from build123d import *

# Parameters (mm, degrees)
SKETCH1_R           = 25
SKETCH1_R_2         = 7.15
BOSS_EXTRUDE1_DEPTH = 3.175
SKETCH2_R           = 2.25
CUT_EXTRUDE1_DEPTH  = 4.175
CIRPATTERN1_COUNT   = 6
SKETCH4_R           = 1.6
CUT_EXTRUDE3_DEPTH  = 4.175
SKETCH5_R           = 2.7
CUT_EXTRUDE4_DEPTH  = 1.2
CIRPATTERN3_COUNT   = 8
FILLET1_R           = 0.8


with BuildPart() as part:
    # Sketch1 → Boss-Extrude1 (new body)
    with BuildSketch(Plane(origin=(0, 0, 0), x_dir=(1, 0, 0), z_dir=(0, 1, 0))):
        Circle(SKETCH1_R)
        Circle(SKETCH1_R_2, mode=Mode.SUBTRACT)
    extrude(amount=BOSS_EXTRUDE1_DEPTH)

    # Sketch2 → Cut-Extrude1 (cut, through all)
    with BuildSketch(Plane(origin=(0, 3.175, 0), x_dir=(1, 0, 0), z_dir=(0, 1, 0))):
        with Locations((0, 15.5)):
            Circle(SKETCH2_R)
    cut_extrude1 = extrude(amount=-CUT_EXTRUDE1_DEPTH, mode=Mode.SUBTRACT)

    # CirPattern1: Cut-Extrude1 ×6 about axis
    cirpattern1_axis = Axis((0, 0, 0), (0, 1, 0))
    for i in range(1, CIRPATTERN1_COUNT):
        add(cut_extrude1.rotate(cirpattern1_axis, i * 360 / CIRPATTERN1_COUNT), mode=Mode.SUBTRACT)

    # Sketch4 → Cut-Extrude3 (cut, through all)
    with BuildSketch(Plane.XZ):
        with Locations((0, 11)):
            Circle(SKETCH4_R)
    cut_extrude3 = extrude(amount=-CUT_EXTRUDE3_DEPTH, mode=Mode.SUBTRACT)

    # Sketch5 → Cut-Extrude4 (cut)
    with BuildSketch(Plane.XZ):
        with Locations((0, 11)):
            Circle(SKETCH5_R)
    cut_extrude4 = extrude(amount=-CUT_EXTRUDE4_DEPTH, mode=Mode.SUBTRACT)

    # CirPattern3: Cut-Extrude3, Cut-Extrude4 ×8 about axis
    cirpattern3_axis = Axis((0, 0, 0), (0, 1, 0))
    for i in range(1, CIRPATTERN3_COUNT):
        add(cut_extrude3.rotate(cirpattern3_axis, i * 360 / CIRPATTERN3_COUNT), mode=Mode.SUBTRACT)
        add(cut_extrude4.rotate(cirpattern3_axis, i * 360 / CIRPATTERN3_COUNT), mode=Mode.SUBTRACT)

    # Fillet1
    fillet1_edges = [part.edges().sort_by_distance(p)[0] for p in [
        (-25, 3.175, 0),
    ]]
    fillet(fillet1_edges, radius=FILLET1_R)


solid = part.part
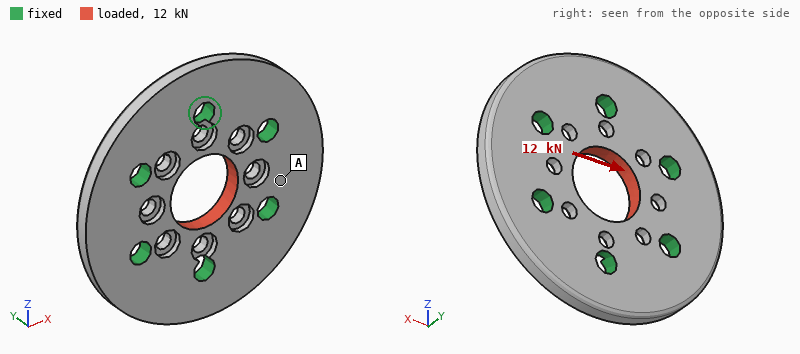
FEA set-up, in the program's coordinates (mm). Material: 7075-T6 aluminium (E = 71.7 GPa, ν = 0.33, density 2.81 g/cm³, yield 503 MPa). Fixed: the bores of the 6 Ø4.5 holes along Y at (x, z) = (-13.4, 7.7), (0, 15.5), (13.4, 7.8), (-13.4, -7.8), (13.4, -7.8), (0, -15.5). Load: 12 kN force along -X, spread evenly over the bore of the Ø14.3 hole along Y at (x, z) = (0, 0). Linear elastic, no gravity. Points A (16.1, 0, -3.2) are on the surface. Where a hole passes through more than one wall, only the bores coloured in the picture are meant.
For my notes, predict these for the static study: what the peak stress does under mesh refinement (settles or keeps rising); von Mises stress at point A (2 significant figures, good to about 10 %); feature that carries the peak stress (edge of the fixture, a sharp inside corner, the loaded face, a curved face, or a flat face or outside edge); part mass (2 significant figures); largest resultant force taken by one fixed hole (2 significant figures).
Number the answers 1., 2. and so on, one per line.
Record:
1. keeps rising
2. 31 MPa
3. a sharp inside corner
4. 14 g
5. 2.6 kN
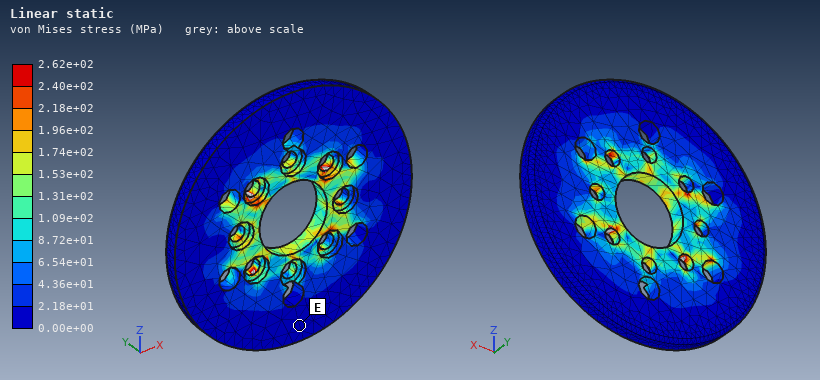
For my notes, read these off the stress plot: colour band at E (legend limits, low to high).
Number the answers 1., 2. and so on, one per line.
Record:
1. 0.00e+00 to 2.18e+01 MPa
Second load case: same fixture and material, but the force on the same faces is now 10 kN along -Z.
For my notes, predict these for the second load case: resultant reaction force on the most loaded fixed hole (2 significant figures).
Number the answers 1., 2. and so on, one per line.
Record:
1. 2.4 kN
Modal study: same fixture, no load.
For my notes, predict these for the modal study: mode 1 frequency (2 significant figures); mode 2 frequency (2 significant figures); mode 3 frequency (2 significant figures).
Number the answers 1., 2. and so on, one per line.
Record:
1. 25 kHz
2. 26 kHz
3. 26 kHz
